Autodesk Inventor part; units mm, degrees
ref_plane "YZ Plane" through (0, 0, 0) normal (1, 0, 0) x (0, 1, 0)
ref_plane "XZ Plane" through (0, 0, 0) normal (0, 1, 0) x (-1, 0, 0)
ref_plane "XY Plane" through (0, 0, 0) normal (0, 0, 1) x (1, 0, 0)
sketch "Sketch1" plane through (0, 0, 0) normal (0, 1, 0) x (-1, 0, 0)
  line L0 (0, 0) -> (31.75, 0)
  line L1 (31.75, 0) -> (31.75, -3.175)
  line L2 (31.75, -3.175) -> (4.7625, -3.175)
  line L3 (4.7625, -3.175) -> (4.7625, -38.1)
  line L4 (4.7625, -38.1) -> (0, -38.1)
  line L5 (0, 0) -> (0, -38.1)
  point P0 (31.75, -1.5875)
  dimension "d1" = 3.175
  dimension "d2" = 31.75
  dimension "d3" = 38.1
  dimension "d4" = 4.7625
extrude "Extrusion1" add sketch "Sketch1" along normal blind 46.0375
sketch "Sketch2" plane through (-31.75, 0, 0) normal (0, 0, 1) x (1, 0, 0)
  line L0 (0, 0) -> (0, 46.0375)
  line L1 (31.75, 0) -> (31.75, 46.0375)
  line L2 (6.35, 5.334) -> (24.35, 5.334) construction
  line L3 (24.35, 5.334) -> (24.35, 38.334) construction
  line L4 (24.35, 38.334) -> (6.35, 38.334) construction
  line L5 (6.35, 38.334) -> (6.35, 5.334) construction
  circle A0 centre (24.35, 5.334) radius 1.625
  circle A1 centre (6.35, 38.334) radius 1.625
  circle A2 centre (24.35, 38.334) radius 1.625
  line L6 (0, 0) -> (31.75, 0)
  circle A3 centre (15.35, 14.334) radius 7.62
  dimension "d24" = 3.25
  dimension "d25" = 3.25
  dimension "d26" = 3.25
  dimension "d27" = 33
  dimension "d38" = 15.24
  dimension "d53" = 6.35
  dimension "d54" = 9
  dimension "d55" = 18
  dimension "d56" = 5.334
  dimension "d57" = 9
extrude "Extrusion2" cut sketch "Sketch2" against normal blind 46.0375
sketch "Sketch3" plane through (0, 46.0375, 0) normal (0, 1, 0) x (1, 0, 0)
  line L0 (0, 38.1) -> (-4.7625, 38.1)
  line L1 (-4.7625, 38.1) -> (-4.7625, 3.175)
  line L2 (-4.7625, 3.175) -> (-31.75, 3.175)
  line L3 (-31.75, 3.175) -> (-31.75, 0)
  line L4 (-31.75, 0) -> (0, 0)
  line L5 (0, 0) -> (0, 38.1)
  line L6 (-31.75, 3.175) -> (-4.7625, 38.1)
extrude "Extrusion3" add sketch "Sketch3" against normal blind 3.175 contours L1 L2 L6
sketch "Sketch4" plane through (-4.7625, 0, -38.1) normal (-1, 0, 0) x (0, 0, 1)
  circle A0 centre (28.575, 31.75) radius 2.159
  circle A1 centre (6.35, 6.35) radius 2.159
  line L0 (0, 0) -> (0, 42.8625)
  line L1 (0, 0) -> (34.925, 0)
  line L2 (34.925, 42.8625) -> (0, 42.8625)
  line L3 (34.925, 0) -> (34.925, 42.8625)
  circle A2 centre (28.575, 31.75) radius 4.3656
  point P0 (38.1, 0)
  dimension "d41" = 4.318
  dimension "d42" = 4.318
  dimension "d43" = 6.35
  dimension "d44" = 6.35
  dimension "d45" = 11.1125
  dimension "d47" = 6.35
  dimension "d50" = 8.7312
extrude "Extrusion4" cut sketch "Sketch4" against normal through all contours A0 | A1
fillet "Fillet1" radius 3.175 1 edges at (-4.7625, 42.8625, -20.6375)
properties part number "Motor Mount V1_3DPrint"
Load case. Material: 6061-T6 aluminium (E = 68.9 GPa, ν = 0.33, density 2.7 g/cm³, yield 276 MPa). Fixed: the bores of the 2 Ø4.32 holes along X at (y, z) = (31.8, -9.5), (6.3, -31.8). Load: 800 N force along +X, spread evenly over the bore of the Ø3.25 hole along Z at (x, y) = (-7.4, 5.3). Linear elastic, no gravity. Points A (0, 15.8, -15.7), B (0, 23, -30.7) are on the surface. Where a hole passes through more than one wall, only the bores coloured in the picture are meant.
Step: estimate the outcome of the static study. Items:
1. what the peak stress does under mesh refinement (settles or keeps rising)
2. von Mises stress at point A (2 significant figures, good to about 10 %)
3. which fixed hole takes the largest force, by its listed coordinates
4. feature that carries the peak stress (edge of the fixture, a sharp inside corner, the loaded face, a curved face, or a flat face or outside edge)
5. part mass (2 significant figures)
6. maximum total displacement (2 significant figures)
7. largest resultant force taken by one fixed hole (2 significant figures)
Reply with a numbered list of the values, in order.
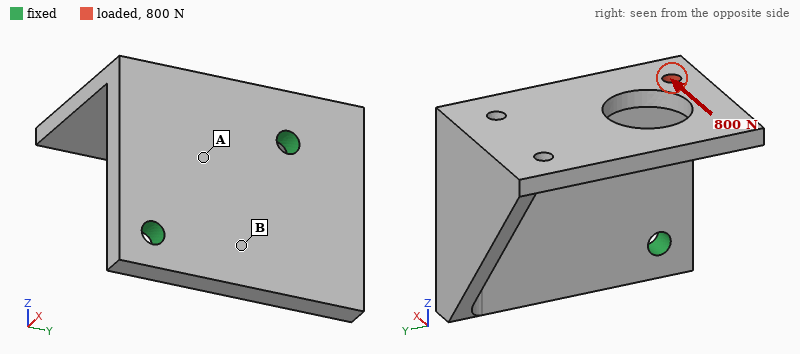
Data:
1. keeps rising
2. 48 MPa
3. (31.8, -9.5)
4. edge of the fixture
5. 35 g
6. 0.23 mm
7. 550 N
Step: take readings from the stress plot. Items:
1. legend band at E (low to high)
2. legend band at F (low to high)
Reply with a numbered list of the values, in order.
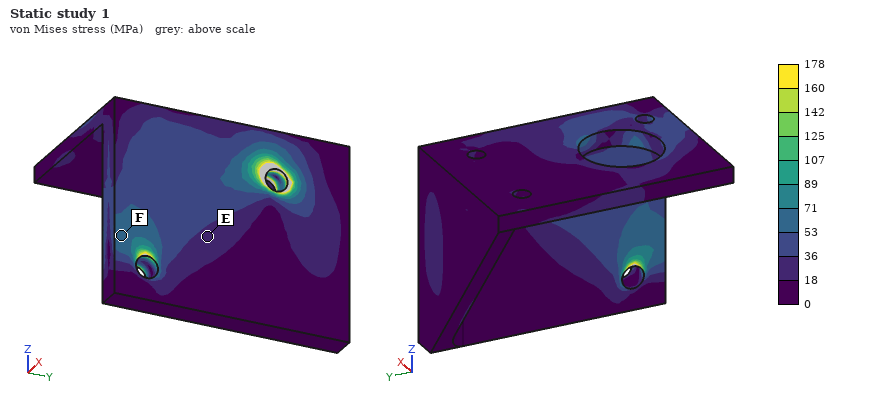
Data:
1. 18 to 36 MPa
2. 53 to 71 MPa
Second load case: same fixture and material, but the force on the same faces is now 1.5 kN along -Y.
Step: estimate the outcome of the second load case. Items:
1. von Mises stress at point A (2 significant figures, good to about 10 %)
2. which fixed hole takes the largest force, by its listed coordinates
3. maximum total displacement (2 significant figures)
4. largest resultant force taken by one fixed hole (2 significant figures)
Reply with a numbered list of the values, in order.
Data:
1. 11 MPa
2. (31.8, -9.5)
3. 70 µm
4. 1.5 kN
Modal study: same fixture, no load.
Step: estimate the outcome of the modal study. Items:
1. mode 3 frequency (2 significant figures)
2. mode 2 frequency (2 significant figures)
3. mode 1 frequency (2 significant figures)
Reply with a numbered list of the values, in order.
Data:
1. 5000 Hz
2. 4200 Hz
3. 3100 Hz
